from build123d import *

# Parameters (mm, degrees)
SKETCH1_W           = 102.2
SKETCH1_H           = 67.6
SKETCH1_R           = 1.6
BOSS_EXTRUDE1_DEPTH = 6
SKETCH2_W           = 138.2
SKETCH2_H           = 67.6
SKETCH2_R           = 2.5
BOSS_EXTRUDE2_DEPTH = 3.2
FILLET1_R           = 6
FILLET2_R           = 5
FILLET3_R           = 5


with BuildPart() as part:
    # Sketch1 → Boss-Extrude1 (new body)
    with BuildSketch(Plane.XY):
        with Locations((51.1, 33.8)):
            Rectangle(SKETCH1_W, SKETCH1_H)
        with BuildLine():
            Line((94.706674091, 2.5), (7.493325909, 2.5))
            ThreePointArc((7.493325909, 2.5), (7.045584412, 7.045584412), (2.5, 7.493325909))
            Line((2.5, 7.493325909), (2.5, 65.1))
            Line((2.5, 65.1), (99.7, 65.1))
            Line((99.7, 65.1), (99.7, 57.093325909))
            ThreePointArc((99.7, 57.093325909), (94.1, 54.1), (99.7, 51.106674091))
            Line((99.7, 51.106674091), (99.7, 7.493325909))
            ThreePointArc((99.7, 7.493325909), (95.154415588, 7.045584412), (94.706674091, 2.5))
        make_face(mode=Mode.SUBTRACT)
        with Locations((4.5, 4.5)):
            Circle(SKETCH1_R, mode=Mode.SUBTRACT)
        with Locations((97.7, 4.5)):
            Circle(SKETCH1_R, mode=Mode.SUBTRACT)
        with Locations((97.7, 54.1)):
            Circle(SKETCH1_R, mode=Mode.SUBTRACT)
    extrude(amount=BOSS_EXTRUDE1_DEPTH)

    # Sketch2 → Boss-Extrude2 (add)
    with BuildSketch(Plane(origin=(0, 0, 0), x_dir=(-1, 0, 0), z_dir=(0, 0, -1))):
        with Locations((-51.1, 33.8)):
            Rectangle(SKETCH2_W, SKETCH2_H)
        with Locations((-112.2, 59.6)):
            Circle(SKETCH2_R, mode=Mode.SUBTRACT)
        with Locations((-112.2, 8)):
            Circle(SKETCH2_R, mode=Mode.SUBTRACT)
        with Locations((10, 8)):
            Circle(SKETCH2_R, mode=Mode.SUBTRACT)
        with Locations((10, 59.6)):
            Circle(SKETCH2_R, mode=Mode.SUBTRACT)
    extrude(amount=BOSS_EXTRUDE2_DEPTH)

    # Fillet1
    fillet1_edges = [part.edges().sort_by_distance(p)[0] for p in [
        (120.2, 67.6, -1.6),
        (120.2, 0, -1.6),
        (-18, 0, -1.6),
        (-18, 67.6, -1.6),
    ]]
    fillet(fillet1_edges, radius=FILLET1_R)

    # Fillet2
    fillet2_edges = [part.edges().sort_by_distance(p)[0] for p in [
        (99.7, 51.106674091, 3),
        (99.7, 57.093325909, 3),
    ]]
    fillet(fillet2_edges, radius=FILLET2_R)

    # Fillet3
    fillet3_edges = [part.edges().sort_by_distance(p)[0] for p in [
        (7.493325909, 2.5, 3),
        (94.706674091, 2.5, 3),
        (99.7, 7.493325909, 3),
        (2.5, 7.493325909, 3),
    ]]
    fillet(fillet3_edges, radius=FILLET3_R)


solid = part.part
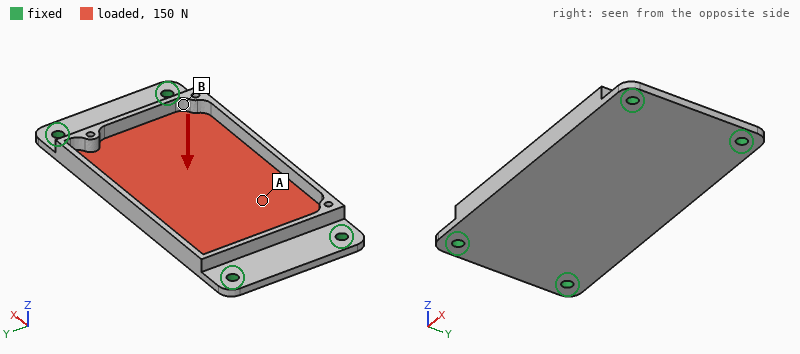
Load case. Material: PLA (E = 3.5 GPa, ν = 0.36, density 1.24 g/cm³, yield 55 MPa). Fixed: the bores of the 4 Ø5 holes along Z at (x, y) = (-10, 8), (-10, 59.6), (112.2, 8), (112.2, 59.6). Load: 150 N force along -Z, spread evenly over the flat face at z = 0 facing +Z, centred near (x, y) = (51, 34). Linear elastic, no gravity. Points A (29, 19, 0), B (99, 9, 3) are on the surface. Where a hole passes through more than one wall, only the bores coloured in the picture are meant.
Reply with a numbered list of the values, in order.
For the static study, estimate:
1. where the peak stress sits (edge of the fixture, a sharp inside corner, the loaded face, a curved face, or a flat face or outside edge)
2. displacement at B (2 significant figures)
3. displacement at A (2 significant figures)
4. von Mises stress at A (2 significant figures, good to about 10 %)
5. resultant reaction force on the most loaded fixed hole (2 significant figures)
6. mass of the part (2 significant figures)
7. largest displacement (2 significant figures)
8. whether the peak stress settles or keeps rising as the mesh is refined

1. edge of the fixture
2. 0.16 mm
3. 0.58 mm
4. 3.0 MPa
5. 60 N
6. 43 g
7. 0.76 mm
8. keeps rising
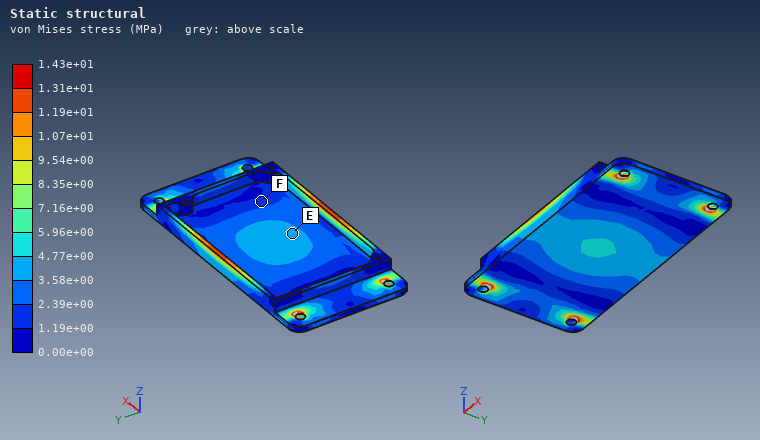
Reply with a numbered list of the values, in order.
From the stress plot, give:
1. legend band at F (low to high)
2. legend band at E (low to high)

1. 1.19e+00 to 2.39e+00 MPa
2. 3.58e+00 to 4.77e+00 MPa
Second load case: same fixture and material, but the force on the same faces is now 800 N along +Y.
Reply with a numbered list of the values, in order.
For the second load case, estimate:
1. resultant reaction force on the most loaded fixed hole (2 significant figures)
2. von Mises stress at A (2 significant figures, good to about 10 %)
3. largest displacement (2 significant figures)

1. 270 N
2. 2.7 MPa
3. 0.28 mm
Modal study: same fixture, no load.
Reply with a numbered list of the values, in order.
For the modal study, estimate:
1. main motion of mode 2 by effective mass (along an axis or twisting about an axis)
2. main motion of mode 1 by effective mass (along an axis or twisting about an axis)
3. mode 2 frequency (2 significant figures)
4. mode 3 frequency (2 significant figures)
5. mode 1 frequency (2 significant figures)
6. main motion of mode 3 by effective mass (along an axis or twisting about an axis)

1. twisting about X
2. along Z
3. 730 Hz
4. 1300 Hz
5. 490 Hz
6. twisting about Y
